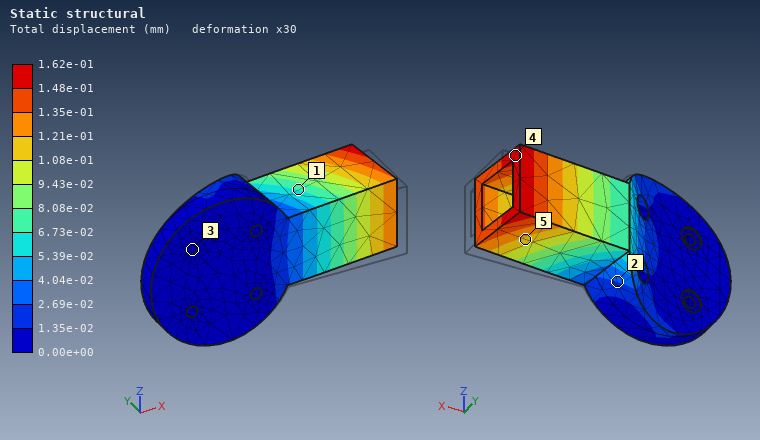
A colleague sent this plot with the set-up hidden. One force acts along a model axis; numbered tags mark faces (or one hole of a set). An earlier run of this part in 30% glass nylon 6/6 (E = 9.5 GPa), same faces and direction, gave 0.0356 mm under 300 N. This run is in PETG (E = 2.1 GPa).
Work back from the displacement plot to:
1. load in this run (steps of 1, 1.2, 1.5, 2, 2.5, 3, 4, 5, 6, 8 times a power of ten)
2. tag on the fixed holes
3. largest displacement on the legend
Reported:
300 N
3
1.62e-01 mm
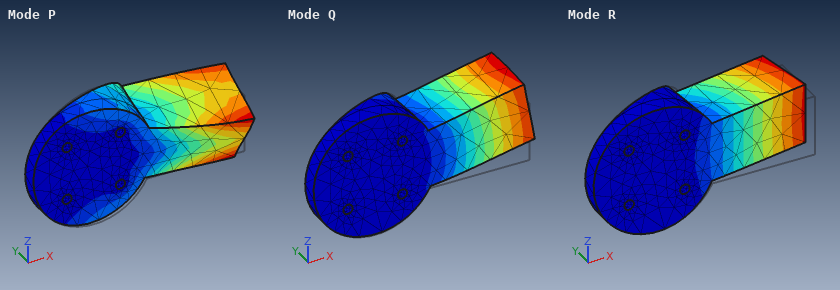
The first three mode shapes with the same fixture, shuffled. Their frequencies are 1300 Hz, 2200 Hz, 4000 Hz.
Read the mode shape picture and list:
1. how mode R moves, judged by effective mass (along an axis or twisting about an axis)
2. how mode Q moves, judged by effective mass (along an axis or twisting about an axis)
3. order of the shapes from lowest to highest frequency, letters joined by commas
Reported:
along Y
along Z
R, Q, P
